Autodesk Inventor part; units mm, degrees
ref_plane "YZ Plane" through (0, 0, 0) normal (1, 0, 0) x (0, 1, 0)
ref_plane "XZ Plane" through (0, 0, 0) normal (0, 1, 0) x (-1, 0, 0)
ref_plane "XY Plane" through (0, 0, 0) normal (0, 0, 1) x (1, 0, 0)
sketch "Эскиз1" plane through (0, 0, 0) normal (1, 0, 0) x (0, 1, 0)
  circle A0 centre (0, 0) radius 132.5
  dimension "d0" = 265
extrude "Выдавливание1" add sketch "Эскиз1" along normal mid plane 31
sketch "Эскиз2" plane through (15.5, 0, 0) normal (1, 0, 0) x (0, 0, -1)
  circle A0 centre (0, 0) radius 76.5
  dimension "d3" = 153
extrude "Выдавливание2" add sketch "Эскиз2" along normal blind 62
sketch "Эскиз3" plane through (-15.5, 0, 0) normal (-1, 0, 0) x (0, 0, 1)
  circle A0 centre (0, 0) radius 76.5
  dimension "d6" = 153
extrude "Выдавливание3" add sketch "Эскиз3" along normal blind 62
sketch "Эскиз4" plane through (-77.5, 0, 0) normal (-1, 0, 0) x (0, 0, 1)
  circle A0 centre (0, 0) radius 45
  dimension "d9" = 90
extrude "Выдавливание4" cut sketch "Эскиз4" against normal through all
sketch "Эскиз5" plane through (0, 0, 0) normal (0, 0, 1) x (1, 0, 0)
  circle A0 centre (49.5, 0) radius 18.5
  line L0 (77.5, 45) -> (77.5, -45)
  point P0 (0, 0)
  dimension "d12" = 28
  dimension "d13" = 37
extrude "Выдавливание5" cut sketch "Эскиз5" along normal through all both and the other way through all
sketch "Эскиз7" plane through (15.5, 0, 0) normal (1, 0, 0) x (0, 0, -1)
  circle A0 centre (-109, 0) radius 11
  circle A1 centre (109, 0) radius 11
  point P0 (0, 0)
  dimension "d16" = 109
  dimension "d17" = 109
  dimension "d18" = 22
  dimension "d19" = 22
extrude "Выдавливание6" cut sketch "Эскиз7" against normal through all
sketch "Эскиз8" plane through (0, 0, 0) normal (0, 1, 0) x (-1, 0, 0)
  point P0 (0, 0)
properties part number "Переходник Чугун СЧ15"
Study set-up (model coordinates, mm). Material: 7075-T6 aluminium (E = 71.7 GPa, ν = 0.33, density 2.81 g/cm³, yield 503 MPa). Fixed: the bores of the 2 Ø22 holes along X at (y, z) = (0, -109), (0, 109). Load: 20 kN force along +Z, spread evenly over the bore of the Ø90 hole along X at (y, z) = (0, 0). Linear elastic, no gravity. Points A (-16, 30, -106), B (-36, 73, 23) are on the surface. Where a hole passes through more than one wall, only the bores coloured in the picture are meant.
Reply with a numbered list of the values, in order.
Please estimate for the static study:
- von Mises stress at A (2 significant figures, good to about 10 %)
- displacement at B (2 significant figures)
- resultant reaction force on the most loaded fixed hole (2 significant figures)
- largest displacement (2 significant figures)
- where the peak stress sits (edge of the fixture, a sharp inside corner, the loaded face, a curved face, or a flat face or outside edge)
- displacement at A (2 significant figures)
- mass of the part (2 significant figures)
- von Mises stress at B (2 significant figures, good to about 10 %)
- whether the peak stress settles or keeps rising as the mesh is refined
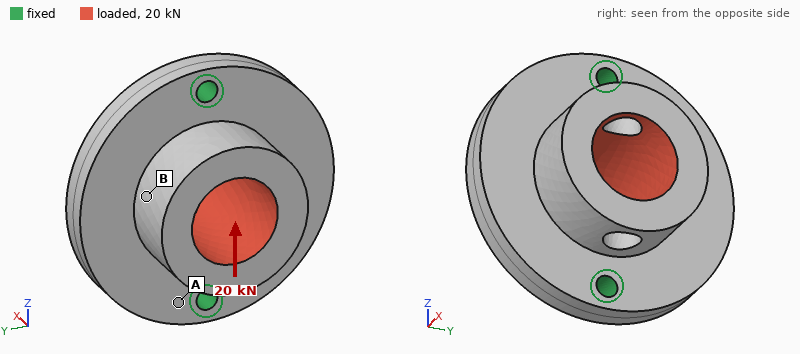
1. 1.8 MPa
2. 4.4 µm
3. 10 kN
4. 6.0 µm
5. edge of the fixture
6. 2.0 µm
7. 8.2 kg
8. 0.82 MPa
9. keeps rising
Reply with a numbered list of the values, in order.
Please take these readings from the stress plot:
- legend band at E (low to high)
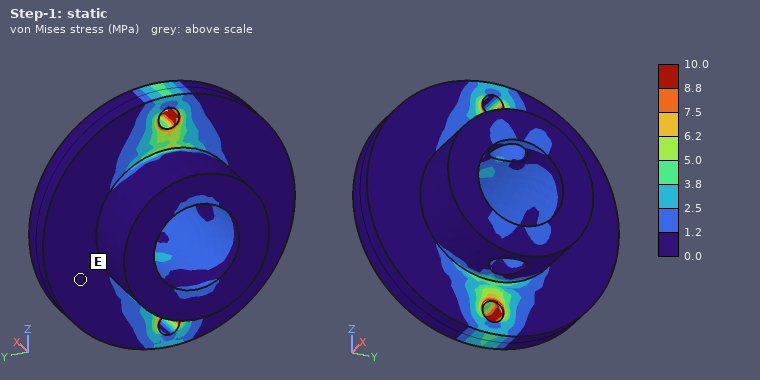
1. 0.0 to 1.2 MPa
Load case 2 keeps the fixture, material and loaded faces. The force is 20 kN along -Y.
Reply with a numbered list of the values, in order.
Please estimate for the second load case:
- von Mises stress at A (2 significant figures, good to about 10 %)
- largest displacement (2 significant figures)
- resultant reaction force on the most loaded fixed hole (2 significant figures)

1. 3.9 MPa
2. 10 µm
3. 10 kN
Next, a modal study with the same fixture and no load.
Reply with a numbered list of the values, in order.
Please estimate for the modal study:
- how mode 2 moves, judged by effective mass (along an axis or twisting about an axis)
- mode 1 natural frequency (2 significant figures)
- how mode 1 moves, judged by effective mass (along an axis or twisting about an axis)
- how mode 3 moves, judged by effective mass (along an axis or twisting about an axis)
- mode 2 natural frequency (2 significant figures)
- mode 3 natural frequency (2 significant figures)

1. along X
2. 960 Hz
3. twisting about Z
4. twisting about Y
5. 2000 Hz
6. 3500 Hz
